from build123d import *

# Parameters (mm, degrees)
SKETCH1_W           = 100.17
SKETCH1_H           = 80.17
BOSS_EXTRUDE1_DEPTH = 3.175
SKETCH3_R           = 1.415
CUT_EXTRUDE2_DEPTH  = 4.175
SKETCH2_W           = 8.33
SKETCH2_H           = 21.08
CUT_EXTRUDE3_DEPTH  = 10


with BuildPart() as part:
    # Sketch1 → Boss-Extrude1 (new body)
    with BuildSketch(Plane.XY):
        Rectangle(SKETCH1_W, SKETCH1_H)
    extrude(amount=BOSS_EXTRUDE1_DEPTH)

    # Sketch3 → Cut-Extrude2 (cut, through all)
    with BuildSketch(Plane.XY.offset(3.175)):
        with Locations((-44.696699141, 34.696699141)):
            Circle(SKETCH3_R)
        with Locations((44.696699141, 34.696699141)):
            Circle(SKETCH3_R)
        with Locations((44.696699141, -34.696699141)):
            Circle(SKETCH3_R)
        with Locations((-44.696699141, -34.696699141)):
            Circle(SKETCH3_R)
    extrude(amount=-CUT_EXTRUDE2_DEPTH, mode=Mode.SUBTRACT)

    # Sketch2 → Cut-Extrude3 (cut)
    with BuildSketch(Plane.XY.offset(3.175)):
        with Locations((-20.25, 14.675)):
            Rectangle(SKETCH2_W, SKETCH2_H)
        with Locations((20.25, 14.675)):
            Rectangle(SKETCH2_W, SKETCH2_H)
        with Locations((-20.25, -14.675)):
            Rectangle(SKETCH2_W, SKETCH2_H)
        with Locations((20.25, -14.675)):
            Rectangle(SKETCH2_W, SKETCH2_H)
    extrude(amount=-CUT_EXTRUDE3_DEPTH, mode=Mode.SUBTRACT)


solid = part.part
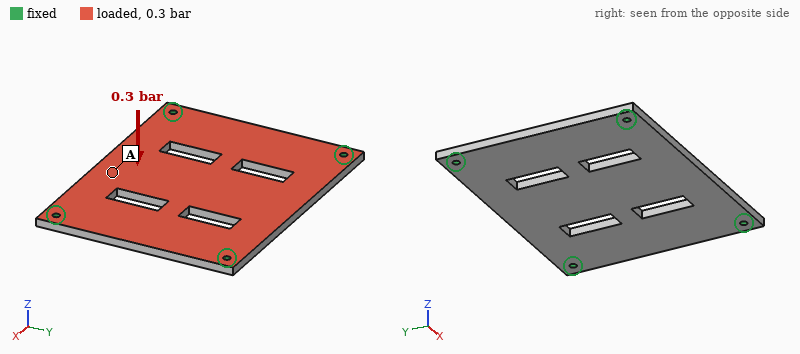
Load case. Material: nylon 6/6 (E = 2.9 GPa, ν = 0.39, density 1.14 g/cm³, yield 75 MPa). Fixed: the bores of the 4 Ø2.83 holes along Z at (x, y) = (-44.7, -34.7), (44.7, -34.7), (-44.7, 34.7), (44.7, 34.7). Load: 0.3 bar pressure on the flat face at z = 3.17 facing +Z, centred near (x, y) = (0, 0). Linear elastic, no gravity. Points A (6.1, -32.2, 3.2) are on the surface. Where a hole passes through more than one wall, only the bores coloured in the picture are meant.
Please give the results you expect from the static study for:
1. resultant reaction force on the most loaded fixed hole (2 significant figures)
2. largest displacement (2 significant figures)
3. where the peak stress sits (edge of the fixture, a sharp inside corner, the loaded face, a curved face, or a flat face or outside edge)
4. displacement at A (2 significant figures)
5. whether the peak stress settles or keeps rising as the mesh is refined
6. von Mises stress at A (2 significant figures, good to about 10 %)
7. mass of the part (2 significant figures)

55 N
1.3 mm
edge of the fixture
1.0 mm
keeps rising
7.2 MPa
26 g
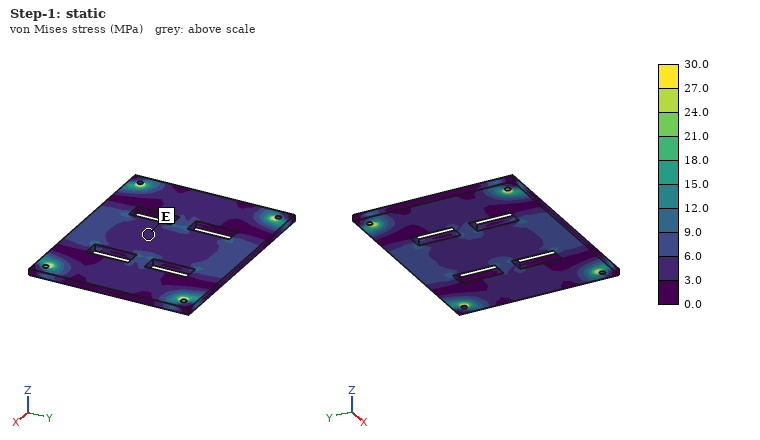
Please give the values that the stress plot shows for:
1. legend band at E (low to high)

3.0 to 6.0 MPa
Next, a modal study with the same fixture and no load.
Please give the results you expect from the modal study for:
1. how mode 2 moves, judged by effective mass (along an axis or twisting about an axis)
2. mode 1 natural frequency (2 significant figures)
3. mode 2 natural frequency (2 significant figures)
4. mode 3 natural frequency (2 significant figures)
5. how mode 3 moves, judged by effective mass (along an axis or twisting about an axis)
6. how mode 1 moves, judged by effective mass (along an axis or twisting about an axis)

twisting about X
470 Hz
750 Hz
980 Hz
twisting about Y
along Z
